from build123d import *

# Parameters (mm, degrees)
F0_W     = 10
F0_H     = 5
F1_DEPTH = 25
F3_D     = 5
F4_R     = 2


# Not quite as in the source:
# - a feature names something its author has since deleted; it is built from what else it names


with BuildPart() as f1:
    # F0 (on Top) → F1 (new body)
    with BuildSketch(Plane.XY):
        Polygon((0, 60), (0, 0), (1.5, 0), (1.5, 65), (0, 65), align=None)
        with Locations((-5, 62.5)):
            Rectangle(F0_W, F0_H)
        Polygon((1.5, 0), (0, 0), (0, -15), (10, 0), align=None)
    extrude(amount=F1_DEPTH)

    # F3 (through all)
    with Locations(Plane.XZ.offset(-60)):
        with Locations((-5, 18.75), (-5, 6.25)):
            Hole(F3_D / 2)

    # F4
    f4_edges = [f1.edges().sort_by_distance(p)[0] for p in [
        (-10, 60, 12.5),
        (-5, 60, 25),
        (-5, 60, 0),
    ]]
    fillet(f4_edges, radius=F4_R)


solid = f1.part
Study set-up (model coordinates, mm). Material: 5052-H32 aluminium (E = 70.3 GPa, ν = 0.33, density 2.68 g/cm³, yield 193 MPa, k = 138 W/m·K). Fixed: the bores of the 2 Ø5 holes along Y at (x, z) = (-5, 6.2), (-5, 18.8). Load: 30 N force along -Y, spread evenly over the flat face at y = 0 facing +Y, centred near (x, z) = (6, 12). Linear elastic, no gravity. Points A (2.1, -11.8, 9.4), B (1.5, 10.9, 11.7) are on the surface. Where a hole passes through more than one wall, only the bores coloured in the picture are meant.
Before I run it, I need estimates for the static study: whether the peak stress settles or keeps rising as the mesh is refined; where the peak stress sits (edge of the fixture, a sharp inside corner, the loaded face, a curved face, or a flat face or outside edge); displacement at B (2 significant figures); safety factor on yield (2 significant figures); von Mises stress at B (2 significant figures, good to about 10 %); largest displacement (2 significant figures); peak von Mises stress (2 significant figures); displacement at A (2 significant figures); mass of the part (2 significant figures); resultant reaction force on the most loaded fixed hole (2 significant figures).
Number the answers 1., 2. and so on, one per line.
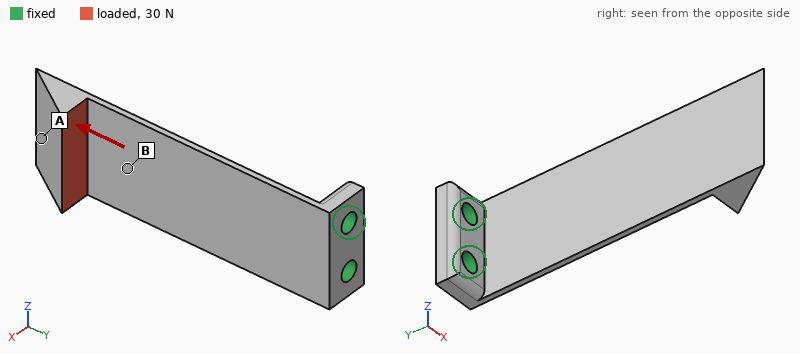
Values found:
1. settles
2. a flat face or outside edge
3. 0.37 mm
4. 11
5. 16 MPa
6. 0.82 mm
7. 17 MPa
8. 0.76 mm
9. 14 g
10. 15 N
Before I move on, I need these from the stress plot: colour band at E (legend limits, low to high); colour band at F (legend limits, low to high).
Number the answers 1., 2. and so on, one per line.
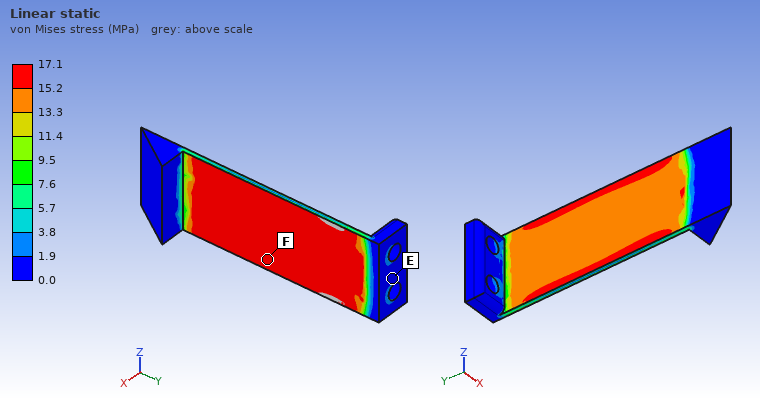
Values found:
1. 0.0 to 1.9 MPa
2. 15.2 to 17.1 MPa
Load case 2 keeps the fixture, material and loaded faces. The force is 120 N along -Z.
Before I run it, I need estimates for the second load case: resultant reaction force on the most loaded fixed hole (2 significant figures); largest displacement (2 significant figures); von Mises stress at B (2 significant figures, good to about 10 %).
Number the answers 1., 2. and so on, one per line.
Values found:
1. 450 N
2. 0.70 mm
3. 57 MPa
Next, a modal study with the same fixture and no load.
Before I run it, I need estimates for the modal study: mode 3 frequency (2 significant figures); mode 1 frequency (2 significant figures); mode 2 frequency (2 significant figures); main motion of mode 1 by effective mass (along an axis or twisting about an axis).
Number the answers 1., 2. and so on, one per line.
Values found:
1. 1300 Hz
2. 150 Hz
3. 910 Hz
4. along X
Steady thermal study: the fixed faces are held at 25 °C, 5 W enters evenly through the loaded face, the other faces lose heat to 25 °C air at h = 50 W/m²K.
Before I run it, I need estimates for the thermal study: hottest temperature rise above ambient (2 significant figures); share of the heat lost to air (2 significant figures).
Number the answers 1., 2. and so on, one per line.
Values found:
1. 30 K
2. 67 %
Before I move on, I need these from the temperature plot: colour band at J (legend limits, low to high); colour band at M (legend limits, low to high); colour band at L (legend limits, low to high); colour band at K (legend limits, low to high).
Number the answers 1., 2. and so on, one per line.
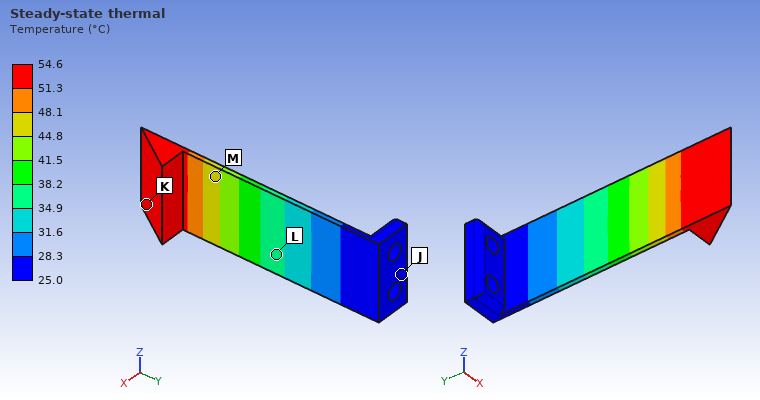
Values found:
1. 25.0 to 28.3 °C
2. 44.8 to 48.1 °C
3. 34.9 to 38.2 °C
4. 51.3 to 54.6 °C
